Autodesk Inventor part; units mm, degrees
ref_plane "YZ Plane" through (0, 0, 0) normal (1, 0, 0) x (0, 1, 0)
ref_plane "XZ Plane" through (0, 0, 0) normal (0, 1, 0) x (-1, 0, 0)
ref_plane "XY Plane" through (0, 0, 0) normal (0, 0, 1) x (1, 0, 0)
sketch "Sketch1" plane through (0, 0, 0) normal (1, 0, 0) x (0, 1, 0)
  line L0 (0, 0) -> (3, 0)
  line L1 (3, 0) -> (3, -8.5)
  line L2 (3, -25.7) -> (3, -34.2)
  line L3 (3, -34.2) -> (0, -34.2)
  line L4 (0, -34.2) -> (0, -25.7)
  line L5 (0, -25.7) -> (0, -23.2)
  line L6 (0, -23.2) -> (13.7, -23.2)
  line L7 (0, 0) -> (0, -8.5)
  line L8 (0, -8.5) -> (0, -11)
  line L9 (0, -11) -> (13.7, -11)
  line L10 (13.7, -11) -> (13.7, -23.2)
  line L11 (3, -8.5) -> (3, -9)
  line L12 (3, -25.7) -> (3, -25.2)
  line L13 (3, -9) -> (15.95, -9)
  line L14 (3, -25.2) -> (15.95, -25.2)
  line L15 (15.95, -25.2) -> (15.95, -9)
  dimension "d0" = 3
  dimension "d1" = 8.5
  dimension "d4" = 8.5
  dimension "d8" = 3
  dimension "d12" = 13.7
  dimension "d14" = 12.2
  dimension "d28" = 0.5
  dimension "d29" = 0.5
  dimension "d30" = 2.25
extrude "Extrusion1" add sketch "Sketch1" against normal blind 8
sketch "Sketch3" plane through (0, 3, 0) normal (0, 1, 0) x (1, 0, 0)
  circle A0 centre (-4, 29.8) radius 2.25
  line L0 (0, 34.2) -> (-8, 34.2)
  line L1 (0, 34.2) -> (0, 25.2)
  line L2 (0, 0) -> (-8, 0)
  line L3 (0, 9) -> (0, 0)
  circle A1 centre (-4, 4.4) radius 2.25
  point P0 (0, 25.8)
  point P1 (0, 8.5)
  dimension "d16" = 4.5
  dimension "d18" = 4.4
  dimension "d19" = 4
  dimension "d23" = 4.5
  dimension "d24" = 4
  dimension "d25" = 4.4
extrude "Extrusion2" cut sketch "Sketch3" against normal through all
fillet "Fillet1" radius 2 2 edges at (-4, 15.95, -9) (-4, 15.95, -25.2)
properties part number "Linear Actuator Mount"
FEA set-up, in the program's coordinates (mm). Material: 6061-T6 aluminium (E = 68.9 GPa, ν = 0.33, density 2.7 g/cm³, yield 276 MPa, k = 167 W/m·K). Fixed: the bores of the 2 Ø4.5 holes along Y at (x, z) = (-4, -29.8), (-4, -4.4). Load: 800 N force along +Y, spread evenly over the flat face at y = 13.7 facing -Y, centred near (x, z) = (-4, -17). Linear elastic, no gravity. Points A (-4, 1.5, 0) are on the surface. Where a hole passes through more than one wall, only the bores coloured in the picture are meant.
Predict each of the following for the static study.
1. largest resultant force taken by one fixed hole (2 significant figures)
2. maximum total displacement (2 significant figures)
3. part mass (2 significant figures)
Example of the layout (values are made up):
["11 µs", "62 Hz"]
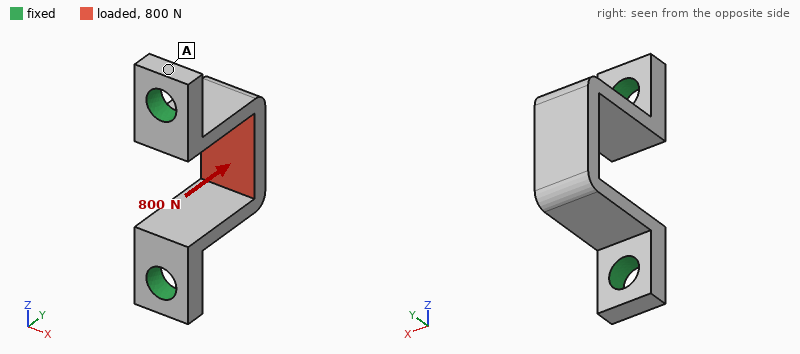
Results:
["410 N", "42 µm", "2.8 g"]
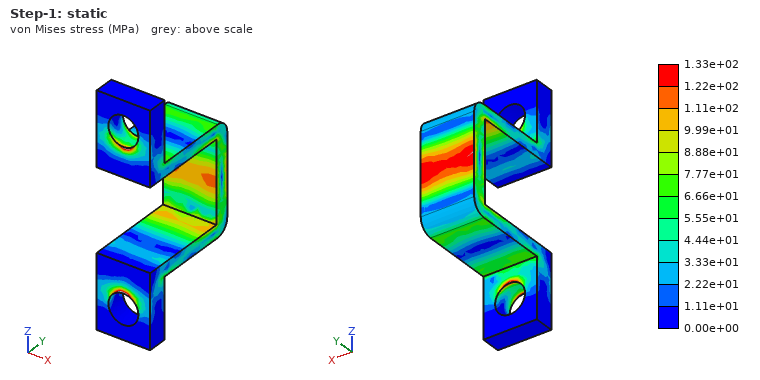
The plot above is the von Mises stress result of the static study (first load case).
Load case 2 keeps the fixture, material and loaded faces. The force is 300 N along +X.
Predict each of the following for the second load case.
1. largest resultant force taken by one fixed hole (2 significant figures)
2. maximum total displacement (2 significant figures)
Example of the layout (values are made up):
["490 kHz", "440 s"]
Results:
["150 N", "77 µm"]
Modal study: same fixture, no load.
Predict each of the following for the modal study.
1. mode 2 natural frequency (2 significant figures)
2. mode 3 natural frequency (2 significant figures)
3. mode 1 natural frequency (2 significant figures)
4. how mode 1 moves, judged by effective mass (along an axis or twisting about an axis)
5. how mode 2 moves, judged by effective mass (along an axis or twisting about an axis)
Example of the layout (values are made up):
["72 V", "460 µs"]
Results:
["9700 Hz", "15 kHz", "8600 Hz", "along Z", "along X"]
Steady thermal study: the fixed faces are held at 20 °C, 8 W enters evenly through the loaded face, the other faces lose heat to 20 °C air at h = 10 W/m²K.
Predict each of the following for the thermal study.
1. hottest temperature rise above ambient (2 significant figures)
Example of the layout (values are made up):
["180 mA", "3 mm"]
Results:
["27 K"]
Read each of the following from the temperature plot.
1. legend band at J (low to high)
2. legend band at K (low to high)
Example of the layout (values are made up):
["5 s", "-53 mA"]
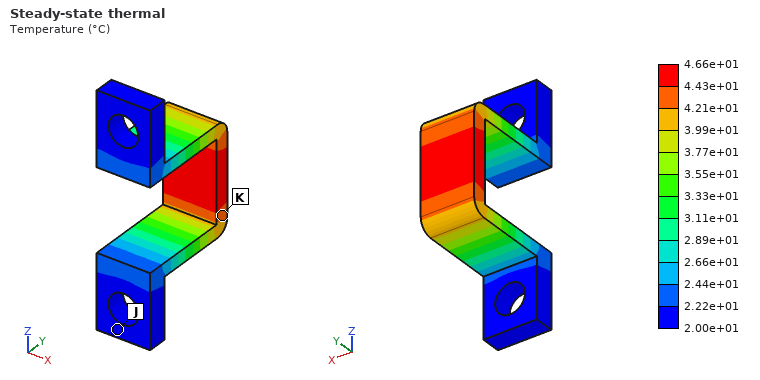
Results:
["2.00e+01 to 2.22e+01 °C", "4.21e+01 to 4.43e+01 °C"]
